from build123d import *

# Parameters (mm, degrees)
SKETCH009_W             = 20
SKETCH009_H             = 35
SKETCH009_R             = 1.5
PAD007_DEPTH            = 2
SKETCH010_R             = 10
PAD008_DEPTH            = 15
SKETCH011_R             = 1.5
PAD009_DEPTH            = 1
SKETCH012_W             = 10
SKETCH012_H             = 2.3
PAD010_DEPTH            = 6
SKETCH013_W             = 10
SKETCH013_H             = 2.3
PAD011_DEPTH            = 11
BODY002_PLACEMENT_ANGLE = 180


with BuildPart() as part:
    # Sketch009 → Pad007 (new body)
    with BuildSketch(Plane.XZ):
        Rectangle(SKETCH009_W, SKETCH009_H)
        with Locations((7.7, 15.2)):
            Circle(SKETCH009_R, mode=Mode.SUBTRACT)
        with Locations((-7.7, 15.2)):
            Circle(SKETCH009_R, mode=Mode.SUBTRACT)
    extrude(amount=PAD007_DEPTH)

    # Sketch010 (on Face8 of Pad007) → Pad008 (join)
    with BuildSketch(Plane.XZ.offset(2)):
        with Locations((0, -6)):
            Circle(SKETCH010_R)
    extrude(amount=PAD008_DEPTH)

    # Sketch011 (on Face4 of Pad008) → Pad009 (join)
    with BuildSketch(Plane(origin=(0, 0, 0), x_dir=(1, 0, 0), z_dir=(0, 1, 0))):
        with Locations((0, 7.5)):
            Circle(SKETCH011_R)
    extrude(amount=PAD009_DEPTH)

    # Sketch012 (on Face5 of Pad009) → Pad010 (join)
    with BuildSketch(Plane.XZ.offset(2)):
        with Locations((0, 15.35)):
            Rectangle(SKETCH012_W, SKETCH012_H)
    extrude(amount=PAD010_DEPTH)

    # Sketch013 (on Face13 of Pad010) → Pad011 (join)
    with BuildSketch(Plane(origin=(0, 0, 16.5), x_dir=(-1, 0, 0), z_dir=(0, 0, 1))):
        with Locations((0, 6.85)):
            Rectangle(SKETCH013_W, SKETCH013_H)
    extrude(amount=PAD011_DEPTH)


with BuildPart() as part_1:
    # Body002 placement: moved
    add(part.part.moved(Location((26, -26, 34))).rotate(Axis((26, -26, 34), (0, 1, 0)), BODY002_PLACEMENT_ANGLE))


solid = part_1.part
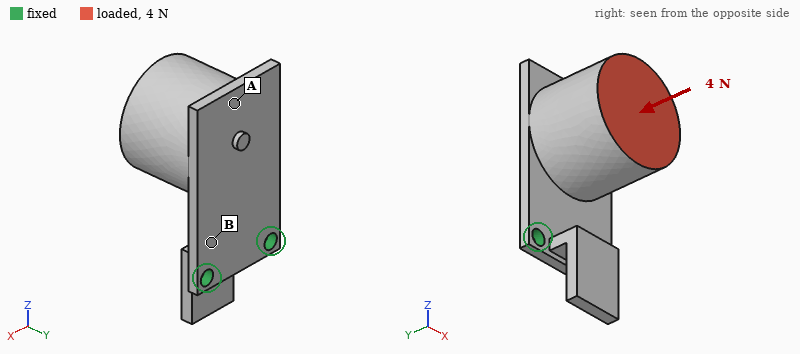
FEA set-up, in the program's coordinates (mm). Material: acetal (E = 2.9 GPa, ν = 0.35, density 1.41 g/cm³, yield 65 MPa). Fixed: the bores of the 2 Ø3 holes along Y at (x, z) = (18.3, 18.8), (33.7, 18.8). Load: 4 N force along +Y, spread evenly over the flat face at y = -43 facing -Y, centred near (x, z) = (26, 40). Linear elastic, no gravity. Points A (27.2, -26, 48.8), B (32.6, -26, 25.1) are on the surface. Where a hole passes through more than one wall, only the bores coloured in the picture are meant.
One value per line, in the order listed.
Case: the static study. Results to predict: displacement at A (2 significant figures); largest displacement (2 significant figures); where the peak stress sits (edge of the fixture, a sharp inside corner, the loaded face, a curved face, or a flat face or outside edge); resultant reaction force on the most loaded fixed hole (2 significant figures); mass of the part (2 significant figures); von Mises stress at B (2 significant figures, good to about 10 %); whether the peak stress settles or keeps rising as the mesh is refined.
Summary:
0.44 mm
0.54 mm
edge of the fixture
2.0 N
9.1 g
4.3 MPa
keeps rising
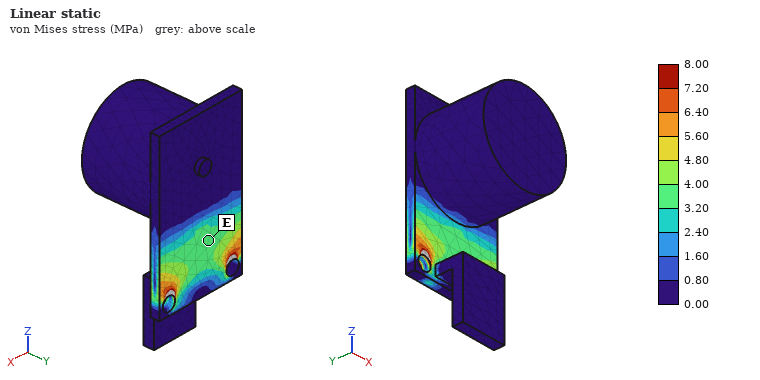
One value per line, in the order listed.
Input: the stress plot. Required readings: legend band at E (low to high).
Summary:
3.20 to 4.00 MPa
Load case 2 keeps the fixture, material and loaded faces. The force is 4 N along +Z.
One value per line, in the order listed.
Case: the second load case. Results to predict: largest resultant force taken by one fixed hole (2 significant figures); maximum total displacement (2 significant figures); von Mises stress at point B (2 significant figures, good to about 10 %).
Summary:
2.3 N
0.58 mm
4.5 MPa
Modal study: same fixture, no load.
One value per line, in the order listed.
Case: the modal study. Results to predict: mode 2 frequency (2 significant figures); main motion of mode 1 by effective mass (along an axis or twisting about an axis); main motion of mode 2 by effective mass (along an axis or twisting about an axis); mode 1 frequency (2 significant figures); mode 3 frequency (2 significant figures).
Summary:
560 Hz
along Y
along X
180 Hz
1400 Hz
